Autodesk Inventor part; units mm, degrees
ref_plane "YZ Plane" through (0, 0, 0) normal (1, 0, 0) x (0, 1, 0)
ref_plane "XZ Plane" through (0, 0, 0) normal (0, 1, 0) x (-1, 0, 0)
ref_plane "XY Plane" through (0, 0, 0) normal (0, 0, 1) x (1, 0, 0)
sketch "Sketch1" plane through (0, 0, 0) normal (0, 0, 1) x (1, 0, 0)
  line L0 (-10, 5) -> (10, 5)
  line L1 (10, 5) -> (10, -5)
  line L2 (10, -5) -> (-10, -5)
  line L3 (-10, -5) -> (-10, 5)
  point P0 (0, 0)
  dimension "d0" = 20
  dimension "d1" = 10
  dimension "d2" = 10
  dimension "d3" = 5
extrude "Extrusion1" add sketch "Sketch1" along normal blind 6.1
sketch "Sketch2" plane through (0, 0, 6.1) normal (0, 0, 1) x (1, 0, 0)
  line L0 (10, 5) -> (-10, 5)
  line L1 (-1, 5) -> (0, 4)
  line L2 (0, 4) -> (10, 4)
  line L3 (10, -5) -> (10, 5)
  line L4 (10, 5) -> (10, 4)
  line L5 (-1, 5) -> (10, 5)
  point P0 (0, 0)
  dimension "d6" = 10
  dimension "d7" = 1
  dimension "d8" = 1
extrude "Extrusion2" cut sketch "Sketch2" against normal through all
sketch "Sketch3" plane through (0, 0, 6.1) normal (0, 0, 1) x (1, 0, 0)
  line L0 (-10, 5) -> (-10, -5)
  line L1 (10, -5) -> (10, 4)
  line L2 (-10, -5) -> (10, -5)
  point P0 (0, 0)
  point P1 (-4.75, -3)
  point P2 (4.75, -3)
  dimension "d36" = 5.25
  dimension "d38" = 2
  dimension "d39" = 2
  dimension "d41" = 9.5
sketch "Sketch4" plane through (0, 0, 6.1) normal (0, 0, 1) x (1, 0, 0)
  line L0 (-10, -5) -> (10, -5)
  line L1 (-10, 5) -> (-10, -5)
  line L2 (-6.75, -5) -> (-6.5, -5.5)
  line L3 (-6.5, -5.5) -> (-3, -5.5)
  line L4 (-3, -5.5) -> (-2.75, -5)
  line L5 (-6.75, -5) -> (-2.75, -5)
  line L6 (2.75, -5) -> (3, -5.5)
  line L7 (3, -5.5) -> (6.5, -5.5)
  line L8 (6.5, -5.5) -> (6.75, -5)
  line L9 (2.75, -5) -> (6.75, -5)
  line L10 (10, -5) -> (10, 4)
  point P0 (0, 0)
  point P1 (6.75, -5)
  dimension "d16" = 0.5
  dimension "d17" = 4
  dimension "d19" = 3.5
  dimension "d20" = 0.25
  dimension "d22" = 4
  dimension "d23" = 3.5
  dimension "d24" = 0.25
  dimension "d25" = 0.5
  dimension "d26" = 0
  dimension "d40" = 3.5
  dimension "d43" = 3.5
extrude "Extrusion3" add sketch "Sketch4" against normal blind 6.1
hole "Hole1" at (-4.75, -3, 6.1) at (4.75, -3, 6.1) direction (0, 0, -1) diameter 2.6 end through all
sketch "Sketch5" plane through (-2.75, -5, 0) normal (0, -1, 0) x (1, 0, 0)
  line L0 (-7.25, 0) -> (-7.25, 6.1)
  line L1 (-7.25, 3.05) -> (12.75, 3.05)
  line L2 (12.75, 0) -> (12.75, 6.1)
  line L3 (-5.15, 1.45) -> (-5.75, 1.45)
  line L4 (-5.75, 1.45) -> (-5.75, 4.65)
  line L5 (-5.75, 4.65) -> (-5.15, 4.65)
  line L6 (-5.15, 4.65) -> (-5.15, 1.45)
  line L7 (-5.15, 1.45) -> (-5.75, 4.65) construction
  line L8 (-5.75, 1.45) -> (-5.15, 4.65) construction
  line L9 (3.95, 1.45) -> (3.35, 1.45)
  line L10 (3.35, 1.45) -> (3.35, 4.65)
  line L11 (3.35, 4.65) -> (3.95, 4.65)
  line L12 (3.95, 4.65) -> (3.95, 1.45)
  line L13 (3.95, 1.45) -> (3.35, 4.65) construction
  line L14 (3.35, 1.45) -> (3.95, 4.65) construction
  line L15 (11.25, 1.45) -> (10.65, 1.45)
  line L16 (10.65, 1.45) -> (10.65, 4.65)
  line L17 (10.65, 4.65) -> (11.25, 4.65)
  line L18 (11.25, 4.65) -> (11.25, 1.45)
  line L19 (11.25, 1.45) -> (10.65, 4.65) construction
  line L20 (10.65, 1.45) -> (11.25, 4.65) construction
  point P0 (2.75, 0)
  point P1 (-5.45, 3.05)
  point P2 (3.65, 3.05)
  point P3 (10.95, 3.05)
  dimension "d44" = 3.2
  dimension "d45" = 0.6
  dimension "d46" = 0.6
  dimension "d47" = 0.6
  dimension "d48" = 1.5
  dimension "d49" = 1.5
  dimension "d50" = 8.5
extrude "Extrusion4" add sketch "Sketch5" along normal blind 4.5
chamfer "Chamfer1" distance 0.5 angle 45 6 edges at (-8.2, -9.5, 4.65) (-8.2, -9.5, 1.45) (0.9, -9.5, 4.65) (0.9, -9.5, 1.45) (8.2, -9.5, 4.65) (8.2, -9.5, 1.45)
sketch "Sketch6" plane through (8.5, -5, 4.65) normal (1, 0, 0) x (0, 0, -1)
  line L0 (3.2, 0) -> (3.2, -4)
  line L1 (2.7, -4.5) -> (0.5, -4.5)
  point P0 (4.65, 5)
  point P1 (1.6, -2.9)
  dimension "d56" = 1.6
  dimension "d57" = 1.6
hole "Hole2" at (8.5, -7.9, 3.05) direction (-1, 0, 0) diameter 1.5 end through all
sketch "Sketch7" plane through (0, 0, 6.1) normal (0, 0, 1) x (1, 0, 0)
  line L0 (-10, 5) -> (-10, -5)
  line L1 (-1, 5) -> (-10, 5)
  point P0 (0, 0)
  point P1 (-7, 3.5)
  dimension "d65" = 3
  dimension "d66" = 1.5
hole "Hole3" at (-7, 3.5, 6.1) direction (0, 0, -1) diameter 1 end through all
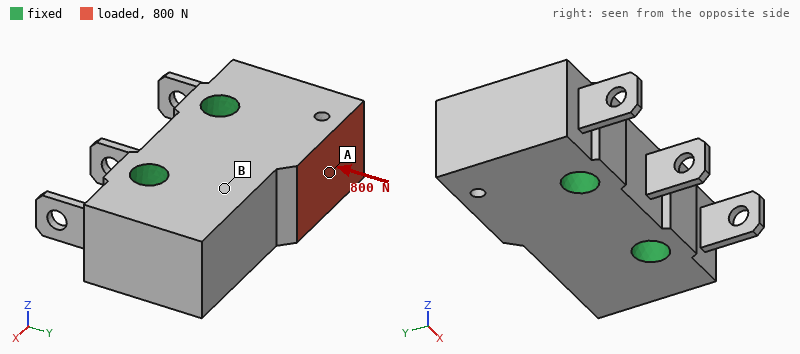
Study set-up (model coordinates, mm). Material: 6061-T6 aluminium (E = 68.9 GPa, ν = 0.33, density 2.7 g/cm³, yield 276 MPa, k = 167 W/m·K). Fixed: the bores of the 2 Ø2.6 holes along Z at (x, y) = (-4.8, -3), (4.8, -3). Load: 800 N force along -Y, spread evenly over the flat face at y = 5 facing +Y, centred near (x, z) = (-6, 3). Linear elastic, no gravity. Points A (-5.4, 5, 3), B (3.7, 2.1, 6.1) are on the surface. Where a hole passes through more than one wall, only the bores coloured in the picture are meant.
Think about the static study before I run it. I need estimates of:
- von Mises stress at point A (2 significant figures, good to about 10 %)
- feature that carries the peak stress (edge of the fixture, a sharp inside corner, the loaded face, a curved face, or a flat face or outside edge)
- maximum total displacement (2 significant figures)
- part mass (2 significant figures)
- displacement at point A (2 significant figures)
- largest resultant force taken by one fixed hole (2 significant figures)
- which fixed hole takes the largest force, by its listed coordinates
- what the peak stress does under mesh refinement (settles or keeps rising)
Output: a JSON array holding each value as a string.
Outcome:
["19 MPa", "edge of the fixture", "3.6 µm", "3.1 g", "2.6 µm", "790 N", "(-4.8, -3)", "keeps rising"]
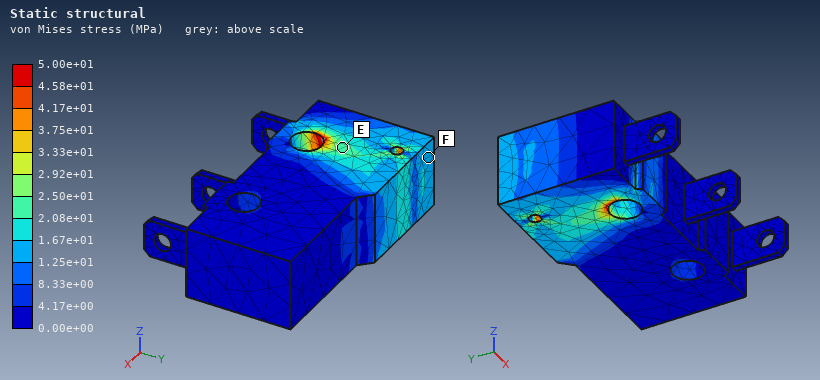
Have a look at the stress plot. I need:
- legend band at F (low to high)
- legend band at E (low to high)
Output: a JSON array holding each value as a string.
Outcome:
["1.25e+01 to 1.67e+01 MPa", "2.08e+01 to 2.50e+01 MPa"]
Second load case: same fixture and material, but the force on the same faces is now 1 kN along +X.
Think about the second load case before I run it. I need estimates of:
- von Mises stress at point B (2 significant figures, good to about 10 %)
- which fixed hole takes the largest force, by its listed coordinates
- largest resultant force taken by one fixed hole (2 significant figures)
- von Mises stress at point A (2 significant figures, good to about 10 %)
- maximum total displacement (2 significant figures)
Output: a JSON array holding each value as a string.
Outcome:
["18 MPa", "(4.8, -3)", "860 N", "48 MPa", "12 µm"]
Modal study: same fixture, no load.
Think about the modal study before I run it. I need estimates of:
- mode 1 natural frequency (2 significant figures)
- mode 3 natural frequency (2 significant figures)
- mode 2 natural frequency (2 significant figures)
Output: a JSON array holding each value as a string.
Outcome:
["25 kHz", "25 kHz", "25 kHz"]
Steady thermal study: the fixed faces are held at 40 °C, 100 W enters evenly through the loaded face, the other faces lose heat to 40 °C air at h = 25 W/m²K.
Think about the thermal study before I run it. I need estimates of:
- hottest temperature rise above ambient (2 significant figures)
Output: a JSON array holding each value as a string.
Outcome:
["80 K"]
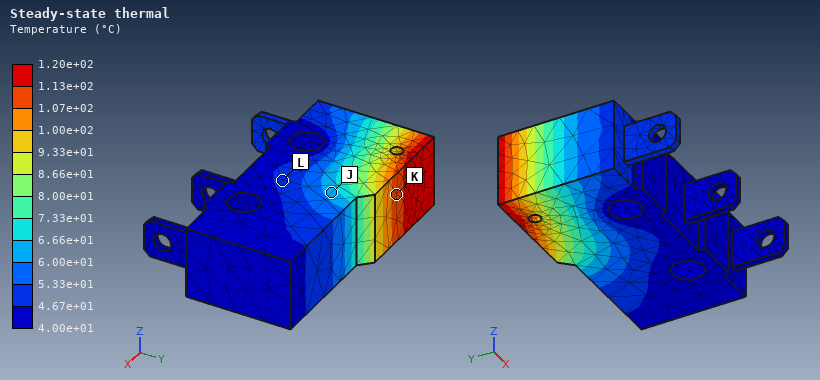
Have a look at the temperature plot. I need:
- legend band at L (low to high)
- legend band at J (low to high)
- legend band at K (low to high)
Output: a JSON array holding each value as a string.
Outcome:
["4.67e+01 to 5.33e+01 °C", "6.00e+01 to 6.66e+01 °C", "1.07e+02 to 1.13e+02 °C"]
